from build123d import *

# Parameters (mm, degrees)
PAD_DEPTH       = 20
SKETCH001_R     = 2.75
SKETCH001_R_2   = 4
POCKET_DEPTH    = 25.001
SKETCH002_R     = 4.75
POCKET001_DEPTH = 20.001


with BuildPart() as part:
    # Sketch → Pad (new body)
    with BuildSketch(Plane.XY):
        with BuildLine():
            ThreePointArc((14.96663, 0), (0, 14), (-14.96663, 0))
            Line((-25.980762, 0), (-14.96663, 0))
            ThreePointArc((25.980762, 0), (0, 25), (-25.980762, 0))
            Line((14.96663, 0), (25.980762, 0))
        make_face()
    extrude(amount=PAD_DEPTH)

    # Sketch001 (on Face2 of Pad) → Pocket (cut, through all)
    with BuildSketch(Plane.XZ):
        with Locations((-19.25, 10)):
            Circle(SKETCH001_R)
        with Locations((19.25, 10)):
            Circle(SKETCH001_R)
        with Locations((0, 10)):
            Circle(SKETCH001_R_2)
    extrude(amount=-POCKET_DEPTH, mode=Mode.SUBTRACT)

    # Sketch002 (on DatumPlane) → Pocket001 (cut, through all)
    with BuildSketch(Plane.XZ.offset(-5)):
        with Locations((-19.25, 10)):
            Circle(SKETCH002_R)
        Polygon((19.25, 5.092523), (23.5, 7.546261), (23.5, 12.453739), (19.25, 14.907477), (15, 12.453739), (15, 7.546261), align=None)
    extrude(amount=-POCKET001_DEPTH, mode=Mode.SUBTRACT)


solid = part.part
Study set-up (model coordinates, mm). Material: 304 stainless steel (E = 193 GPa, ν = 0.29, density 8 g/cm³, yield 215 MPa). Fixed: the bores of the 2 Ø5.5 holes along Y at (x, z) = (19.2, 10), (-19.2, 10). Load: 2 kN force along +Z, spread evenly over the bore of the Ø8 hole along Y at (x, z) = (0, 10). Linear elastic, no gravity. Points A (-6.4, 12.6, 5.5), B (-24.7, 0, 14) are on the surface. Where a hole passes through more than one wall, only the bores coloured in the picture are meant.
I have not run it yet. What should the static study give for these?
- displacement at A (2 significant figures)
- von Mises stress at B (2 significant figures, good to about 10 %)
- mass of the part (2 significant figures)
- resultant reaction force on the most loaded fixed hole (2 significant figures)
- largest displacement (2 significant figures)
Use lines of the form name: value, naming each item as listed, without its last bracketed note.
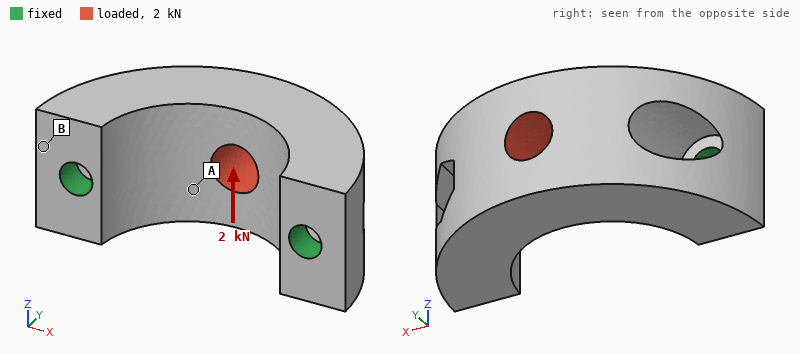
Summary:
displacement at A: 12 µm
von Mises stress at B: 39 MPa
mass of the part: 92 g
resultant reaction force on the most loaded fixed hole: 1.0 kN
largest displacement: 24 µm
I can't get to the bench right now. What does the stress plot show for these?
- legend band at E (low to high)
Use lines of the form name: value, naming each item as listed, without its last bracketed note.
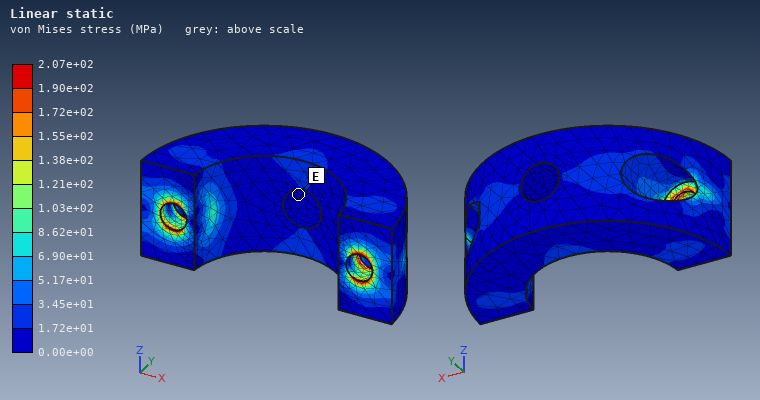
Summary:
legend band at E: 0.00e+00 to 1.72e+01 MPa
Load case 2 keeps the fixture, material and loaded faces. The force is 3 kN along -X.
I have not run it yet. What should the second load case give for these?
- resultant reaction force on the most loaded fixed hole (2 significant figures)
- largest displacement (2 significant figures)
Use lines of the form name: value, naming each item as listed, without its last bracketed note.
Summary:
resultant reaction force on the most loaded fixed hole: 1.9 kN
largest displacement: 5.6 µm
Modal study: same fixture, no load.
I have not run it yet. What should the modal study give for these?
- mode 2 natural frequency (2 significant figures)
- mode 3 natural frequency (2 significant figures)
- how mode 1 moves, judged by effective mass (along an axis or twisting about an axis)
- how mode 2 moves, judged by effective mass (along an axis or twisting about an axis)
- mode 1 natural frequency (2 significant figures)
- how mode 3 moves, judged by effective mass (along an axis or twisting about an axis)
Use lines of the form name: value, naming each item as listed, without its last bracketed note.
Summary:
mode 2 natural frequency: 16 kHz
mode 3 natural frequency: 18 kHz
how mode 1 moves, judged by effective mass: along Z
how mode 2 moves, judged by effective mass: along X
mode 1 natural frequency: 7300 Hz
how mode 3 moves, judged by effective mass: twisting about Y
